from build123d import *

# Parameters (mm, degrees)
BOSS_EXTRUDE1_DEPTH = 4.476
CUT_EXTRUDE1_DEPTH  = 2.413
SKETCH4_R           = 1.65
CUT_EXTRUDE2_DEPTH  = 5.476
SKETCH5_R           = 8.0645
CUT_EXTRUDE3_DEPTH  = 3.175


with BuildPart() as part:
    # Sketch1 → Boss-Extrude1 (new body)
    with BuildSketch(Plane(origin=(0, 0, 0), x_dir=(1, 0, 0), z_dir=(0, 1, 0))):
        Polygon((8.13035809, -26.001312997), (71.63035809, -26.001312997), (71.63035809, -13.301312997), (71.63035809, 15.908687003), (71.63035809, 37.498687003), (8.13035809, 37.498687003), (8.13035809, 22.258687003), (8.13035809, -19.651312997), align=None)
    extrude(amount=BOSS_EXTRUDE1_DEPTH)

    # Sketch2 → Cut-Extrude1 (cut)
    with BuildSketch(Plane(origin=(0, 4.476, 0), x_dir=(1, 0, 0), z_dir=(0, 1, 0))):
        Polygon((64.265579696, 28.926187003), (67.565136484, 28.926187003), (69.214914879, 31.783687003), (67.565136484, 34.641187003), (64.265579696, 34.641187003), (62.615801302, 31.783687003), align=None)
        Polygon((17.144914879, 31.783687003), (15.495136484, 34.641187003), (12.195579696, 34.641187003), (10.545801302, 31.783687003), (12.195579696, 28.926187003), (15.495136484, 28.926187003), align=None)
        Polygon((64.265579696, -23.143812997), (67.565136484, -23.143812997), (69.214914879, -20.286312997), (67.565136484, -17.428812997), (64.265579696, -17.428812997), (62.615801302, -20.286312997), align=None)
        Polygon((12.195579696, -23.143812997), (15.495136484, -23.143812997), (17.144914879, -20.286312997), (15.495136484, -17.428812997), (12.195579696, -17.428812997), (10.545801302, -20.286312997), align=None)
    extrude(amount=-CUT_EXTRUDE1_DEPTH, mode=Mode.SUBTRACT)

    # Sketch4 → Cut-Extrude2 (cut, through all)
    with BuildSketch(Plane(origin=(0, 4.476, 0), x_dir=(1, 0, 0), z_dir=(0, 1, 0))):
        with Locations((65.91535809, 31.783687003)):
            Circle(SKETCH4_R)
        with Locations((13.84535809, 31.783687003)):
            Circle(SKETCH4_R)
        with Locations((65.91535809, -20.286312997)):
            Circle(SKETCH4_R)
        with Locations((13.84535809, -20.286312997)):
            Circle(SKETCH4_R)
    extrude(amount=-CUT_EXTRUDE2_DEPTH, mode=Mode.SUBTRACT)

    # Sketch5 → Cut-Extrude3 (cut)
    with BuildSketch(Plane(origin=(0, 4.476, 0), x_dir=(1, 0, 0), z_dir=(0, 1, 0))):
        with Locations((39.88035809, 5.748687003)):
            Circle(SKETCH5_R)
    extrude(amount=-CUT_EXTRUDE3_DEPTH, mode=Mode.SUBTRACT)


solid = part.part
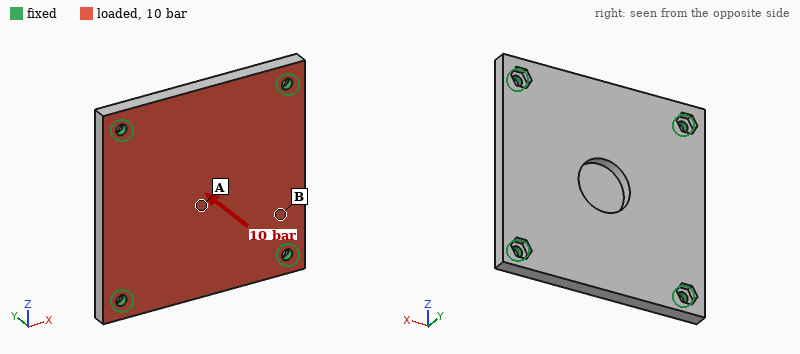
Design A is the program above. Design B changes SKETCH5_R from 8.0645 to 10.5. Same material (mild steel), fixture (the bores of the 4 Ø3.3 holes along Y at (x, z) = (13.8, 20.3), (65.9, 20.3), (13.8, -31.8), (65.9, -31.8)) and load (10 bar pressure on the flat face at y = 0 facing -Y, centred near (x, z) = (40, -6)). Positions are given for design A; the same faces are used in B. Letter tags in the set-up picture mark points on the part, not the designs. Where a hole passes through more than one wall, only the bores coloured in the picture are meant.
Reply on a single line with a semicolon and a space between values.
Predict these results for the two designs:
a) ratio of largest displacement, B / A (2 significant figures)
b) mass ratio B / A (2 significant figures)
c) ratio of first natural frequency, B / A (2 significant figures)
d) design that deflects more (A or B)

1.1; 0.97; 1.0; B
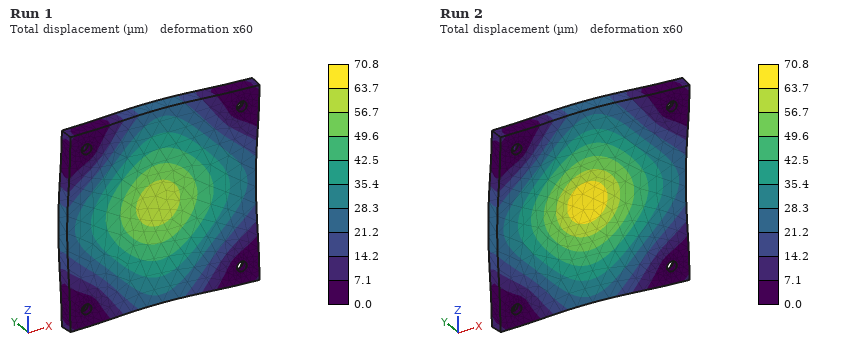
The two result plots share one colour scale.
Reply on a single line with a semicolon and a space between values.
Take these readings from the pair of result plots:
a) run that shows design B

Run 2
